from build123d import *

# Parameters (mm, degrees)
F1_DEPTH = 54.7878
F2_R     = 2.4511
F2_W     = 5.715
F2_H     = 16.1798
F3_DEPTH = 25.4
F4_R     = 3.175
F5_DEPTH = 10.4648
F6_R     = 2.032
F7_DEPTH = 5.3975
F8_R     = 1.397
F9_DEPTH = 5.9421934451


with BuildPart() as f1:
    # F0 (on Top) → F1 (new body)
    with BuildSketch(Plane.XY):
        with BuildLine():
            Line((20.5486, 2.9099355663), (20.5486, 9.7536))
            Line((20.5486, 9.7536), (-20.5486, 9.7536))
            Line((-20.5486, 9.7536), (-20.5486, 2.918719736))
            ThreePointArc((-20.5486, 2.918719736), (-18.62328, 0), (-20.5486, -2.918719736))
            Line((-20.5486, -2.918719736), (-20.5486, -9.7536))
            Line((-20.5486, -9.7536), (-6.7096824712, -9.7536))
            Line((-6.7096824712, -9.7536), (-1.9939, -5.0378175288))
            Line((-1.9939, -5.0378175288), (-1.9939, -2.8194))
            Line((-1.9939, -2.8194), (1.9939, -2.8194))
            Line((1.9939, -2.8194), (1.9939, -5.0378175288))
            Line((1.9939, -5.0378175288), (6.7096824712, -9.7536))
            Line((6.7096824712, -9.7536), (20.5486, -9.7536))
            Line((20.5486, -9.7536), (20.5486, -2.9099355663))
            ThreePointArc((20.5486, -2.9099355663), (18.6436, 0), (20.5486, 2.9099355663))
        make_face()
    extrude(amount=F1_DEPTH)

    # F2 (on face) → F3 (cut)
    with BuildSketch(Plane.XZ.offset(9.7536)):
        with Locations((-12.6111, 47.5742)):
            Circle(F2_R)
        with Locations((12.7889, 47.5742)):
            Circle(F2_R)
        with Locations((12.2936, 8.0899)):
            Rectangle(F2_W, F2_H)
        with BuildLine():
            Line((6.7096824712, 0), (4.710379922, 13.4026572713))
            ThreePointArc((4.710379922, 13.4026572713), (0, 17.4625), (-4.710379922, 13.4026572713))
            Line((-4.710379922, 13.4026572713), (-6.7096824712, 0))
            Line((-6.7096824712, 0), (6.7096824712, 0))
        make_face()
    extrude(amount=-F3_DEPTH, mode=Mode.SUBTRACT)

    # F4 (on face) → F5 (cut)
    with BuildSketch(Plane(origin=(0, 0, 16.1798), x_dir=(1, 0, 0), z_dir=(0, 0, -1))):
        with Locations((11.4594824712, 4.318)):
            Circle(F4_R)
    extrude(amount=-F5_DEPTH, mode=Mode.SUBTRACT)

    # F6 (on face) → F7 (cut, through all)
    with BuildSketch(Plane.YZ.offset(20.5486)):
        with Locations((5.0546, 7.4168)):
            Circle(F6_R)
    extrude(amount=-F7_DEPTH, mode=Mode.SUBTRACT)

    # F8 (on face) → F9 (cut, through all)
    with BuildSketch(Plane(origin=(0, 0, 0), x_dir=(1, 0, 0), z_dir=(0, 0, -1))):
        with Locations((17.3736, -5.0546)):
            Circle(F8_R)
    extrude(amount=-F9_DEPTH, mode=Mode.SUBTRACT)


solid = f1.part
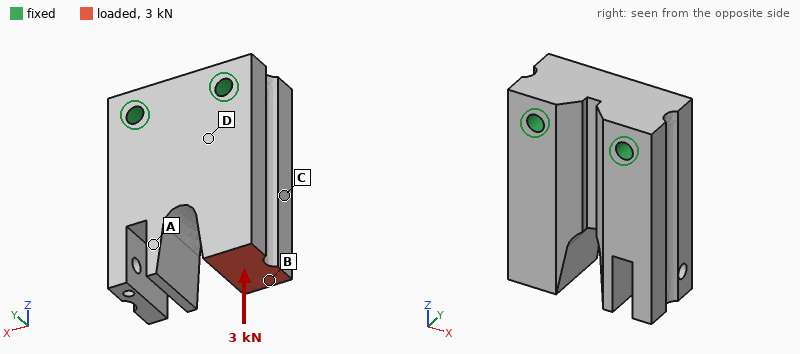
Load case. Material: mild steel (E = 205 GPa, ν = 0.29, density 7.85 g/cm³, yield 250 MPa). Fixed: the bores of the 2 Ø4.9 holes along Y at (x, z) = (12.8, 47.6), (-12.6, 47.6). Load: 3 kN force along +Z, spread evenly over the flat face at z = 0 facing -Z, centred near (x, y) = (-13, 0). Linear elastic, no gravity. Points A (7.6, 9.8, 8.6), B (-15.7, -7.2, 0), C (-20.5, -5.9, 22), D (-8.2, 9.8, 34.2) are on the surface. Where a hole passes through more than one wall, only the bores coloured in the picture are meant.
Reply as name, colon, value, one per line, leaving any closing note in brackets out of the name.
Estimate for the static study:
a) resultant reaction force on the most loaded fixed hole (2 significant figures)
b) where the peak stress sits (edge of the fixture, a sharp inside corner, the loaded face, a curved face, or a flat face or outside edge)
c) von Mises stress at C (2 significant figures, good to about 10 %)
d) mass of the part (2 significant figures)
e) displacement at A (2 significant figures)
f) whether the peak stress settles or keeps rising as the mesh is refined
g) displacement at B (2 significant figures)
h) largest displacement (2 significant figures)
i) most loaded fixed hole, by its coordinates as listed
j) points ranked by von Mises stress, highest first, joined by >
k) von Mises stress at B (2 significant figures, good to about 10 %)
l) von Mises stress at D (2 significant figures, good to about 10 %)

resultant reaction force on the most loaded fixed hole: 3.0 kN
where the peak stress sits: edge of the fixture
von Mises stress at C: 15 MPa
mass of the part: 270 g
displacement at A: 1.1 µm
whether the peak stress settles or keeps rising as the mesh is refined: keeps rising
displacement at B: 4.0 µm
largest displacement: 4.4 µm
most loaded fixed hole, by its coordinates as listed: (-12.6, 47.6)
points ranked by von Mises stress, highest first, joined by >: C > B > D > A
von Mises stress at B: 11 MPa
von Mises stress at D: 6.4 MPa
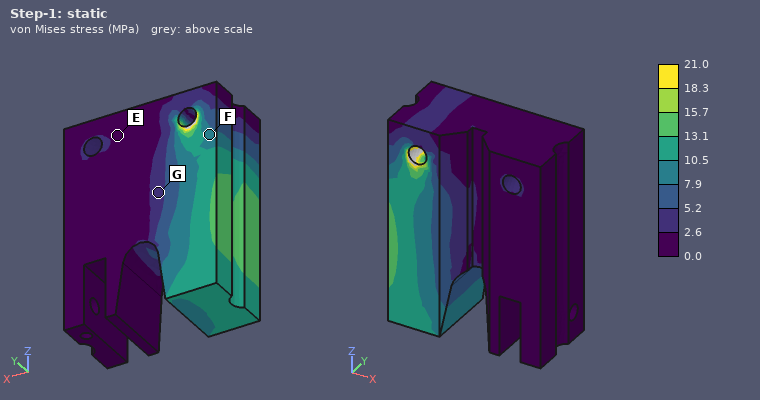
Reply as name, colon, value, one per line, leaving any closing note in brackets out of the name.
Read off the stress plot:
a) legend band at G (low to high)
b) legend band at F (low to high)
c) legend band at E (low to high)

legend band at G: 2.6 to 5.2 MPa
legend band at F: 7.9 to 10.5 MPa
legend band at E: 0.0 to 2.6 MPa
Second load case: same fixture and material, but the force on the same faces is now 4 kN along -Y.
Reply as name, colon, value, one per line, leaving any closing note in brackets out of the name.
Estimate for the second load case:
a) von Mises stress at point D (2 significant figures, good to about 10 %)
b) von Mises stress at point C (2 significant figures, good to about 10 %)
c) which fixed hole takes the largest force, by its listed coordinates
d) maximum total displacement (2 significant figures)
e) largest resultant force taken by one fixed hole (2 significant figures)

von Mises stress at point D: 81 MPa
von Mises stress at point C: 48 MPa
which fixed hole takes the largest force, by its listed coordinates: (-12.6, 47.6)
maximum total displacement: 65 µm
largest resultant force taken by one fixed hole: 3.3 kN
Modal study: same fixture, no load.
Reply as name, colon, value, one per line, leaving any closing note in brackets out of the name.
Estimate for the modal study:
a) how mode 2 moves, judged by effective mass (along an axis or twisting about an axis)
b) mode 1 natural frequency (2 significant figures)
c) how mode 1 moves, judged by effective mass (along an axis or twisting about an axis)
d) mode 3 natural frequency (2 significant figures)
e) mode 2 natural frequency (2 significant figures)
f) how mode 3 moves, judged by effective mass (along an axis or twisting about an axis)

how mode 2 moves, judged by effective mass: along X
mode 1 natural frequency: 7100 Hz
how mode 1 moves, judged by effective mass: along Y
mode 3 natural frequency: 11 kHz
mode 2 natural frequency: 9300 Hz
how mode 3 moves, judged by effective mass: twisting about Z
